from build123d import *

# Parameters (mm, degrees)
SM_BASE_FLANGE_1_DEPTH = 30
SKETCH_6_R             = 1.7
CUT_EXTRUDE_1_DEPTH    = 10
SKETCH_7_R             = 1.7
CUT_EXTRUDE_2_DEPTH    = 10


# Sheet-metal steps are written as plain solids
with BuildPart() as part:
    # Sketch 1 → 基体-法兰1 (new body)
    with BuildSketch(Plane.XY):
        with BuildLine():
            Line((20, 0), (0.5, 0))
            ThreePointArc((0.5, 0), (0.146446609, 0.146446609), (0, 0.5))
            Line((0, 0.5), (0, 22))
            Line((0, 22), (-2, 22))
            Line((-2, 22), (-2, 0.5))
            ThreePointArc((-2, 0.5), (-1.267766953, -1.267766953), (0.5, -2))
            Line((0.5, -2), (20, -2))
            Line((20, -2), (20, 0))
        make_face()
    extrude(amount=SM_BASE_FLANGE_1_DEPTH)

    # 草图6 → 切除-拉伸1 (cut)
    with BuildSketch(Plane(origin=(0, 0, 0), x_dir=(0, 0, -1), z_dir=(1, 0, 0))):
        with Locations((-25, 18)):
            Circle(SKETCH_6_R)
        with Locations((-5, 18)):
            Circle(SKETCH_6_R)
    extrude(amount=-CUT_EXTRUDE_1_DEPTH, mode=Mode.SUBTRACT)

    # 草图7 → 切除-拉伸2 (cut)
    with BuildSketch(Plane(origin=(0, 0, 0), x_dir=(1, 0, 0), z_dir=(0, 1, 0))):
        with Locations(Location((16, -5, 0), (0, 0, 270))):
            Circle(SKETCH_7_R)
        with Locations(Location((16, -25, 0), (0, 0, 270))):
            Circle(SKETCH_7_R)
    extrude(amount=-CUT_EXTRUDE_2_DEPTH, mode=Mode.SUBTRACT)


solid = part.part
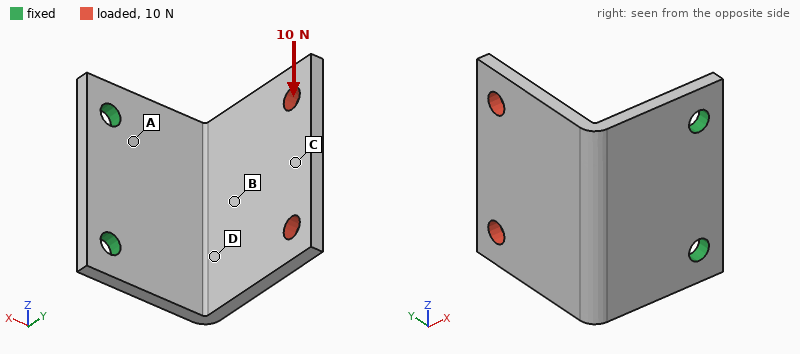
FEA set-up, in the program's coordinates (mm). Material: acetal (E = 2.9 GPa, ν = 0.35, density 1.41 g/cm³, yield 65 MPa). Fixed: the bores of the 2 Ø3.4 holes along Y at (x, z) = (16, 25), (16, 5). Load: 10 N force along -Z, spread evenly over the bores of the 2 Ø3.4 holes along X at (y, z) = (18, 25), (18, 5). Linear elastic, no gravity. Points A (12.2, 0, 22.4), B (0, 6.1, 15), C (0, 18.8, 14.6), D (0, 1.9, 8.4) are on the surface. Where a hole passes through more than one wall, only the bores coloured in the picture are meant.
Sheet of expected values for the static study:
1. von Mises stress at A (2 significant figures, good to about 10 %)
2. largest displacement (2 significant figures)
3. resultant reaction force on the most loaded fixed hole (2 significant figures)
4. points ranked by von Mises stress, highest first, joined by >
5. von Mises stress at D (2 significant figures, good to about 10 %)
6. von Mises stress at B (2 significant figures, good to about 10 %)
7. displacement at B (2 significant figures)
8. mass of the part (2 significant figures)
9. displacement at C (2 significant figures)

4.6 MPa
0.45 mm
13 N
A > D > B > C
3.3 MPa
1.9 MPa
0.12 mm
3.6 g
0.32 mm
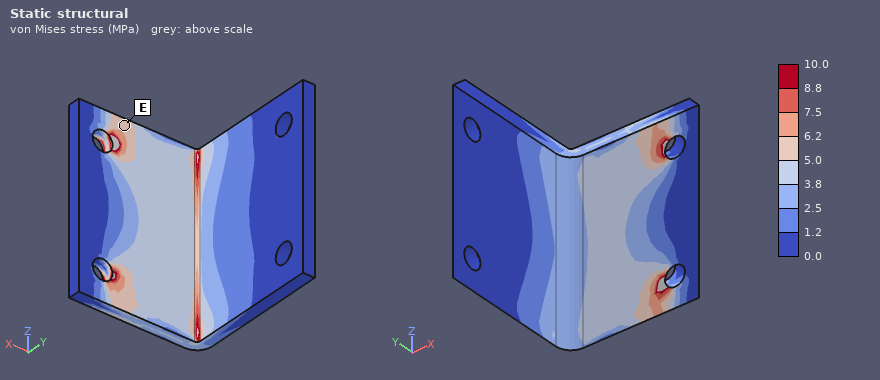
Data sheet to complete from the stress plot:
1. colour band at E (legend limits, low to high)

5.0 to 6.2 MPa
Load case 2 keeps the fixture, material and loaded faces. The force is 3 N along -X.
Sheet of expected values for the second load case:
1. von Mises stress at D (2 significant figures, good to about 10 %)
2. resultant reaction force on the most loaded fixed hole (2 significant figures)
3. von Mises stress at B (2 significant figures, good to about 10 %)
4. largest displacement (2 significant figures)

2.2 MPa
1.6 N
1.6 MPa
0.51 mm
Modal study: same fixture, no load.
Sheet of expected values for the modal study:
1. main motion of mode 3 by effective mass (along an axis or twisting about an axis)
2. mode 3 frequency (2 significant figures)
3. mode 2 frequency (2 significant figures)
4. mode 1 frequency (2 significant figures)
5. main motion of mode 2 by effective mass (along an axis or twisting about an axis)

along Y
1200 Hz
770 Hz
410 Hz
along Z
